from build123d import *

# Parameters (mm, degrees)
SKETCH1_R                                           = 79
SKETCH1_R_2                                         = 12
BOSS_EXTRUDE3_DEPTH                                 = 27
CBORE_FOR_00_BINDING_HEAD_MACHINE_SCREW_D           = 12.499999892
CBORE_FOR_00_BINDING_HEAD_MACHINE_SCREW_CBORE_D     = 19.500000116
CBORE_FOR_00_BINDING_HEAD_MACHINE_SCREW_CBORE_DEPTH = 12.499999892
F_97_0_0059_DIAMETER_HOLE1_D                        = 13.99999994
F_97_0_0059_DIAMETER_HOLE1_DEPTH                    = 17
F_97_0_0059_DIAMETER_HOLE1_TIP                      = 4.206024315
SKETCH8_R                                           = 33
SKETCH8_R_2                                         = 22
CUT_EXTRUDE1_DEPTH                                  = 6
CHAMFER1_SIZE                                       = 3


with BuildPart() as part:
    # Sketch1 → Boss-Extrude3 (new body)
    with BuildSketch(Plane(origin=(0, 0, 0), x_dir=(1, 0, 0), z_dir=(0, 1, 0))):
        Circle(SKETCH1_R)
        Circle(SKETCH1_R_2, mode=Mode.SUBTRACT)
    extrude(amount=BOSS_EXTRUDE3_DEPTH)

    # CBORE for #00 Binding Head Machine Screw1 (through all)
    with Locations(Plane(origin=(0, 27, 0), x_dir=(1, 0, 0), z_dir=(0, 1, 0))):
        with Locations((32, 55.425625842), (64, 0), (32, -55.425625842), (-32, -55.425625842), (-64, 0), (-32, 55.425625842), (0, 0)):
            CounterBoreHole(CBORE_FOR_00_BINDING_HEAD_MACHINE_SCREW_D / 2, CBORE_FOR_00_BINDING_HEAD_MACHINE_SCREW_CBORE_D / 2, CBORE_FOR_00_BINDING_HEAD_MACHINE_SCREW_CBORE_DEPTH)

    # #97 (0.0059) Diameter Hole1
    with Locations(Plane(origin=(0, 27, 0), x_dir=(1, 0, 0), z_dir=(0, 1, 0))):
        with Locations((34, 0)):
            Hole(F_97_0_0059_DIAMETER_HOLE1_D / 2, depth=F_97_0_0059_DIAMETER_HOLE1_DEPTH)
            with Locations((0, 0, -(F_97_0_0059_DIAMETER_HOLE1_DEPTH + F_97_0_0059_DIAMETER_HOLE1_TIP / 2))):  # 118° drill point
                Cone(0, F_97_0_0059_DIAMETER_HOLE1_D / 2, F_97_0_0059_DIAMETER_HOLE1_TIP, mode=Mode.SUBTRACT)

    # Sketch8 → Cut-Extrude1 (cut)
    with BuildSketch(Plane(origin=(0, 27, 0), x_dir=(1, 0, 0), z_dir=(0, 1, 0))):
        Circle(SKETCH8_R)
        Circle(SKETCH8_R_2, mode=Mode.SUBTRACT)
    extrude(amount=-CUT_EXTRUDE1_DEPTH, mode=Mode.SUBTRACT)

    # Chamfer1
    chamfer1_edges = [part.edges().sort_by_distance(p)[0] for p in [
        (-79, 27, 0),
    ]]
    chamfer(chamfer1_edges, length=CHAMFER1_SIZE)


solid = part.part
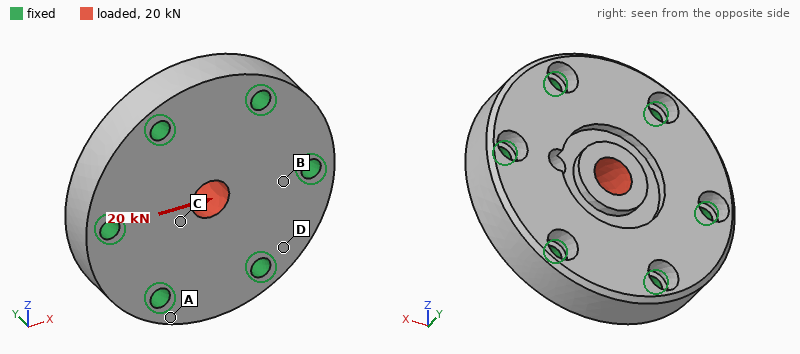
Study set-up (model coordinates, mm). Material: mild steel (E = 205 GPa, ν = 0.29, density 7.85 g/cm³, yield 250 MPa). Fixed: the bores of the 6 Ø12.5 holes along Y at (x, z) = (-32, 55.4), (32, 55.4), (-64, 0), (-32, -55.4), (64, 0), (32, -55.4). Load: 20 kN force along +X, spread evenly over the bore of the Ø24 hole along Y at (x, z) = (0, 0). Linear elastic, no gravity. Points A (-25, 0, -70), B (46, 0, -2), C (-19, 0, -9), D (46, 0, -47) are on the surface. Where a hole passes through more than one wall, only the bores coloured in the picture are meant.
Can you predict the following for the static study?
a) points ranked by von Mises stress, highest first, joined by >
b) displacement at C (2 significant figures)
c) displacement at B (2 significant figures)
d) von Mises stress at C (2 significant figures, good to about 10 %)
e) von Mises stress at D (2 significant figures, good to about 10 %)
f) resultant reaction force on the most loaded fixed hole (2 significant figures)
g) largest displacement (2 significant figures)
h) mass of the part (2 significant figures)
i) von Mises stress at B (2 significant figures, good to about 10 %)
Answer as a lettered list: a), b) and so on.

a) B > C > D > A
b) 1.6 µm
c) 0.68 µm
d) 7.7 MPa
e) 3.8 MPa
f) 5.0 kN
g) 3.3 µm
h) 3.7 kg
i) 11 MPa
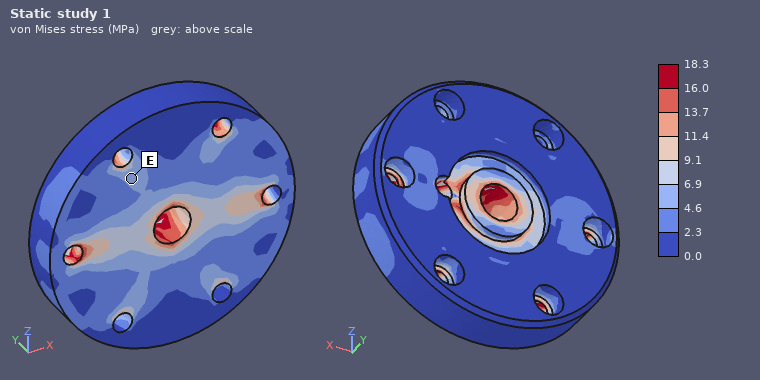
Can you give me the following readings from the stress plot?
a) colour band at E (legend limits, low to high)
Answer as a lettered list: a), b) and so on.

a) 4.6 to 6.9 MPa
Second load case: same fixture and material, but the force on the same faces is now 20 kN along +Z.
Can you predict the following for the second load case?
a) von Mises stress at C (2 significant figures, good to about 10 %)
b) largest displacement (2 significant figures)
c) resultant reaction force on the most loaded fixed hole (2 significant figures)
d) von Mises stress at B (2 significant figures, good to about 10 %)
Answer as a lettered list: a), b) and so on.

a) 5.9 MPa
b) 3.0 µm
c) 4.4 kN
d) 1.6 MPa
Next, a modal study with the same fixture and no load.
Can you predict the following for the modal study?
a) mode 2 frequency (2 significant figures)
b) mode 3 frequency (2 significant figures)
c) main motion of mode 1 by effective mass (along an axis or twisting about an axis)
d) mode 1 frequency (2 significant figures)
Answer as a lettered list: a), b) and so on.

a) 14 kHz
b) 14 kHz
c) along Y
d) 8700 Hz
